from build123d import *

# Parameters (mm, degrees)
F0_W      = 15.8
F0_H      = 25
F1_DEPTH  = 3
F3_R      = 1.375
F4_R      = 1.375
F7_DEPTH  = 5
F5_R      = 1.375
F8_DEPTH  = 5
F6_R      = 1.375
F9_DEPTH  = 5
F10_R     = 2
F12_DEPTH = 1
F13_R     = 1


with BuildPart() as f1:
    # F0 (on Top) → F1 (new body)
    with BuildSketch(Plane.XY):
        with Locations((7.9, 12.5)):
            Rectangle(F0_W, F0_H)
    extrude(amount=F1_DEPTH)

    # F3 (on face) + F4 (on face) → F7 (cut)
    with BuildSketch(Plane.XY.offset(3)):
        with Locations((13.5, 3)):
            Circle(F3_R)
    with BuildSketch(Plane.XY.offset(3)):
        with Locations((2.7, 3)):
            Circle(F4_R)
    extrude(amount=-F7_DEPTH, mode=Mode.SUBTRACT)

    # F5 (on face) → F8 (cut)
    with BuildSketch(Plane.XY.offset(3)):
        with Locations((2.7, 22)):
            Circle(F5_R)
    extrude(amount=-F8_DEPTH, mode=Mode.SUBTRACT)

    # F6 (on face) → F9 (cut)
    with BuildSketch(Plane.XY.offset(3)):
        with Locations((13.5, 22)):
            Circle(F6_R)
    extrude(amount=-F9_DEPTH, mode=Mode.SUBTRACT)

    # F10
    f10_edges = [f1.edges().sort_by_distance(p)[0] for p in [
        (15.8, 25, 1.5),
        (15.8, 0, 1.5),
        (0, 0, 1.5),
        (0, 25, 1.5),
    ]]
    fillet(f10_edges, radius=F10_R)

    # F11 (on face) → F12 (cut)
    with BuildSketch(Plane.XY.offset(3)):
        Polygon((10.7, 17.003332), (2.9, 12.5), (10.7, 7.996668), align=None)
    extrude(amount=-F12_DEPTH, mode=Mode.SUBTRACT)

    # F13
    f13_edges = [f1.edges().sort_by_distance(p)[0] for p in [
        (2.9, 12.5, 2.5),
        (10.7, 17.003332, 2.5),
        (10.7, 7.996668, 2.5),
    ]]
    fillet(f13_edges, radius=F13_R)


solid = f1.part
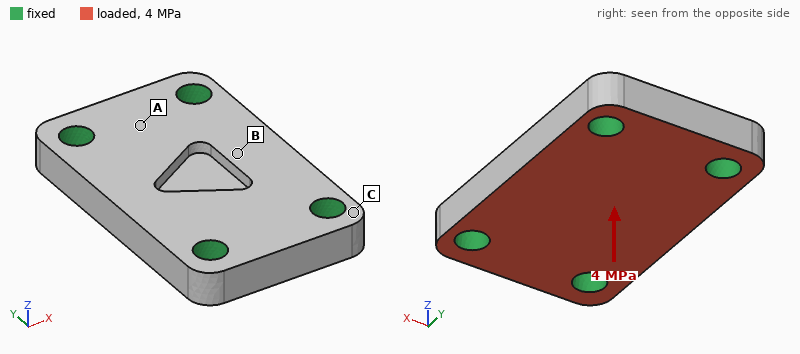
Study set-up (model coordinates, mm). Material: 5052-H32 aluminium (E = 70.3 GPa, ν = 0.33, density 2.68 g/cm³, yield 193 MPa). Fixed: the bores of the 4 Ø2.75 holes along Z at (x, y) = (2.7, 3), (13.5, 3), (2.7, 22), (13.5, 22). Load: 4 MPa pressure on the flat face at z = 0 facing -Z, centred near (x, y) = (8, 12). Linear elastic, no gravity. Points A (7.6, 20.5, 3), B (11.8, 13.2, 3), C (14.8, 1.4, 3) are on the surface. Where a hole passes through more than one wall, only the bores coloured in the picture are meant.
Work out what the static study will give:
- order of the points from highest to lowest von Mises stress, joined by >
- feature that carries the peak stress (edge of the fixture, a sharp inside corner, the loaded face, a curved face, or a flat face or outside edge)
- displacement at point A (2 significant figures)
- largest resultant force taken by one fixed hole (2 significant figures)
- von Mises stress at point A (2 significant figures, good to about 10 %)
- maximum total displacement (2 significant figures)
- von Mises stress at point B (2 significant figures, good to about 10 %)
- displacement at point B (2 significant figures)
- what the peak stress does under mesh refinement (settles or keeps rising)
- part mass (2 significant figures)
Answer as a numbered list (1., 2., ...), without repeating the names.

1. B > A > C
2. edge of the fixture
3. 3.2 µm
4. 380 N
5. 23 MPa
6. 11 µm
7. 41 MPa
8. 10.0 µm
9. keeps rising
10. 2.9 g
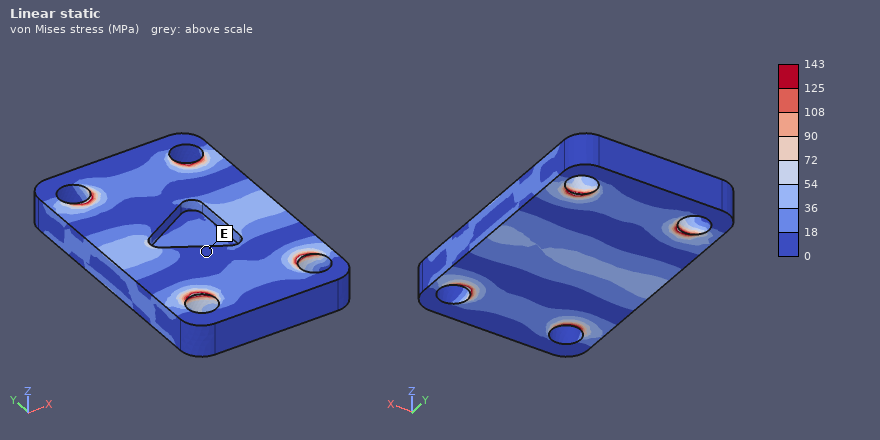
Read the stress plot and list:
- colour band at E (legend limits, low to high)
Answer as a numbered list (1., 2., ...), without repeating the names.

1. 0 to 18 MPa
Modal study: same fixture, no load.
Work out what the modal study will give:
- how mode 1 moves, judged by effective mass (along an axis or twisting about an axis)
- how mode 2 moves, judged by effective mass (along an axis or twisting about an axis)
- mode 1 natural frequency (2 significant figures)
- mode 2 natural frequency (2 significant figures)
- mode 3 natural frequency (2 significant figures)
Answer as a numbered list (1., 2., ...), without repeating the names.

1. along Z
2. twisting about Y
3. 41 kHz
4. 52 kHz
5. 78 kHz
